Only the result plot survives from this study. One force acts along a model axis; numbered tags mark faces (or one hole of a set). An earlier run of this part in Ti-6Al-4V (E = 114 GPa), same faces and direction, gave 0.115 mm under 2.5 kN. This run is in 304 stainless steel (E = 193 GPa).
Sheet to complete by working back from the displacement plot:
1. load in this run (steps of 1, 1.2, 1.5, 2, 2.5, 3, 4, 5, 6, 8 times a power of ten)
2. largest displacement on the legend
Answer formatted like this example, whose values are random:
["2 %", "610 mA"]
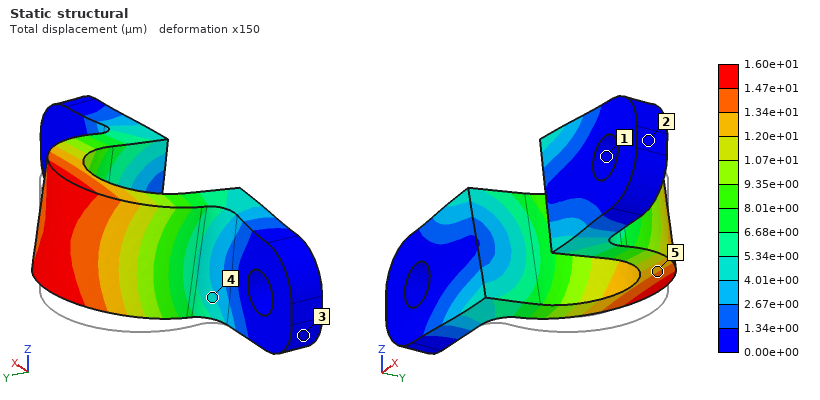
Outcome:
["600 N", "1.60e+01 µm"]
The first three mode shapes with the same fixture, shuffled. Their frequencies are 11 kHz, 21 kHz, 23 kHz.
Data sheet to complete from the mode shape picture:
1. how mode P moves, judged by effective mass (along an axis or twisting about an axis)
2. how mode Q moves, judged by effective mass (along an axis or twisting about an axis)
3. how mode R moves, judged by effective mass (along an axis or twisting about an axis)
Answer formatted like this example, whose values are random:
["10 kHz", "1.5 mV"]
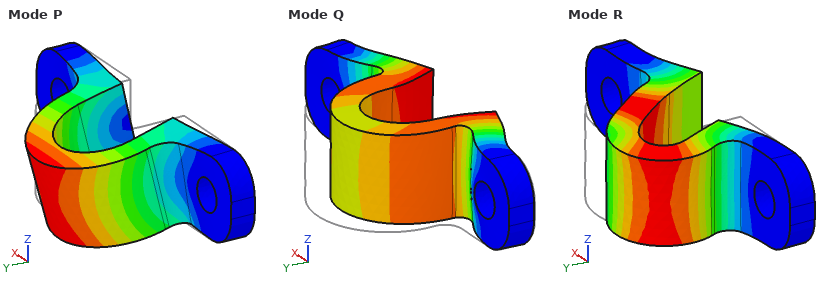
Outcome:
["along Z", "along Y", "along X"]
